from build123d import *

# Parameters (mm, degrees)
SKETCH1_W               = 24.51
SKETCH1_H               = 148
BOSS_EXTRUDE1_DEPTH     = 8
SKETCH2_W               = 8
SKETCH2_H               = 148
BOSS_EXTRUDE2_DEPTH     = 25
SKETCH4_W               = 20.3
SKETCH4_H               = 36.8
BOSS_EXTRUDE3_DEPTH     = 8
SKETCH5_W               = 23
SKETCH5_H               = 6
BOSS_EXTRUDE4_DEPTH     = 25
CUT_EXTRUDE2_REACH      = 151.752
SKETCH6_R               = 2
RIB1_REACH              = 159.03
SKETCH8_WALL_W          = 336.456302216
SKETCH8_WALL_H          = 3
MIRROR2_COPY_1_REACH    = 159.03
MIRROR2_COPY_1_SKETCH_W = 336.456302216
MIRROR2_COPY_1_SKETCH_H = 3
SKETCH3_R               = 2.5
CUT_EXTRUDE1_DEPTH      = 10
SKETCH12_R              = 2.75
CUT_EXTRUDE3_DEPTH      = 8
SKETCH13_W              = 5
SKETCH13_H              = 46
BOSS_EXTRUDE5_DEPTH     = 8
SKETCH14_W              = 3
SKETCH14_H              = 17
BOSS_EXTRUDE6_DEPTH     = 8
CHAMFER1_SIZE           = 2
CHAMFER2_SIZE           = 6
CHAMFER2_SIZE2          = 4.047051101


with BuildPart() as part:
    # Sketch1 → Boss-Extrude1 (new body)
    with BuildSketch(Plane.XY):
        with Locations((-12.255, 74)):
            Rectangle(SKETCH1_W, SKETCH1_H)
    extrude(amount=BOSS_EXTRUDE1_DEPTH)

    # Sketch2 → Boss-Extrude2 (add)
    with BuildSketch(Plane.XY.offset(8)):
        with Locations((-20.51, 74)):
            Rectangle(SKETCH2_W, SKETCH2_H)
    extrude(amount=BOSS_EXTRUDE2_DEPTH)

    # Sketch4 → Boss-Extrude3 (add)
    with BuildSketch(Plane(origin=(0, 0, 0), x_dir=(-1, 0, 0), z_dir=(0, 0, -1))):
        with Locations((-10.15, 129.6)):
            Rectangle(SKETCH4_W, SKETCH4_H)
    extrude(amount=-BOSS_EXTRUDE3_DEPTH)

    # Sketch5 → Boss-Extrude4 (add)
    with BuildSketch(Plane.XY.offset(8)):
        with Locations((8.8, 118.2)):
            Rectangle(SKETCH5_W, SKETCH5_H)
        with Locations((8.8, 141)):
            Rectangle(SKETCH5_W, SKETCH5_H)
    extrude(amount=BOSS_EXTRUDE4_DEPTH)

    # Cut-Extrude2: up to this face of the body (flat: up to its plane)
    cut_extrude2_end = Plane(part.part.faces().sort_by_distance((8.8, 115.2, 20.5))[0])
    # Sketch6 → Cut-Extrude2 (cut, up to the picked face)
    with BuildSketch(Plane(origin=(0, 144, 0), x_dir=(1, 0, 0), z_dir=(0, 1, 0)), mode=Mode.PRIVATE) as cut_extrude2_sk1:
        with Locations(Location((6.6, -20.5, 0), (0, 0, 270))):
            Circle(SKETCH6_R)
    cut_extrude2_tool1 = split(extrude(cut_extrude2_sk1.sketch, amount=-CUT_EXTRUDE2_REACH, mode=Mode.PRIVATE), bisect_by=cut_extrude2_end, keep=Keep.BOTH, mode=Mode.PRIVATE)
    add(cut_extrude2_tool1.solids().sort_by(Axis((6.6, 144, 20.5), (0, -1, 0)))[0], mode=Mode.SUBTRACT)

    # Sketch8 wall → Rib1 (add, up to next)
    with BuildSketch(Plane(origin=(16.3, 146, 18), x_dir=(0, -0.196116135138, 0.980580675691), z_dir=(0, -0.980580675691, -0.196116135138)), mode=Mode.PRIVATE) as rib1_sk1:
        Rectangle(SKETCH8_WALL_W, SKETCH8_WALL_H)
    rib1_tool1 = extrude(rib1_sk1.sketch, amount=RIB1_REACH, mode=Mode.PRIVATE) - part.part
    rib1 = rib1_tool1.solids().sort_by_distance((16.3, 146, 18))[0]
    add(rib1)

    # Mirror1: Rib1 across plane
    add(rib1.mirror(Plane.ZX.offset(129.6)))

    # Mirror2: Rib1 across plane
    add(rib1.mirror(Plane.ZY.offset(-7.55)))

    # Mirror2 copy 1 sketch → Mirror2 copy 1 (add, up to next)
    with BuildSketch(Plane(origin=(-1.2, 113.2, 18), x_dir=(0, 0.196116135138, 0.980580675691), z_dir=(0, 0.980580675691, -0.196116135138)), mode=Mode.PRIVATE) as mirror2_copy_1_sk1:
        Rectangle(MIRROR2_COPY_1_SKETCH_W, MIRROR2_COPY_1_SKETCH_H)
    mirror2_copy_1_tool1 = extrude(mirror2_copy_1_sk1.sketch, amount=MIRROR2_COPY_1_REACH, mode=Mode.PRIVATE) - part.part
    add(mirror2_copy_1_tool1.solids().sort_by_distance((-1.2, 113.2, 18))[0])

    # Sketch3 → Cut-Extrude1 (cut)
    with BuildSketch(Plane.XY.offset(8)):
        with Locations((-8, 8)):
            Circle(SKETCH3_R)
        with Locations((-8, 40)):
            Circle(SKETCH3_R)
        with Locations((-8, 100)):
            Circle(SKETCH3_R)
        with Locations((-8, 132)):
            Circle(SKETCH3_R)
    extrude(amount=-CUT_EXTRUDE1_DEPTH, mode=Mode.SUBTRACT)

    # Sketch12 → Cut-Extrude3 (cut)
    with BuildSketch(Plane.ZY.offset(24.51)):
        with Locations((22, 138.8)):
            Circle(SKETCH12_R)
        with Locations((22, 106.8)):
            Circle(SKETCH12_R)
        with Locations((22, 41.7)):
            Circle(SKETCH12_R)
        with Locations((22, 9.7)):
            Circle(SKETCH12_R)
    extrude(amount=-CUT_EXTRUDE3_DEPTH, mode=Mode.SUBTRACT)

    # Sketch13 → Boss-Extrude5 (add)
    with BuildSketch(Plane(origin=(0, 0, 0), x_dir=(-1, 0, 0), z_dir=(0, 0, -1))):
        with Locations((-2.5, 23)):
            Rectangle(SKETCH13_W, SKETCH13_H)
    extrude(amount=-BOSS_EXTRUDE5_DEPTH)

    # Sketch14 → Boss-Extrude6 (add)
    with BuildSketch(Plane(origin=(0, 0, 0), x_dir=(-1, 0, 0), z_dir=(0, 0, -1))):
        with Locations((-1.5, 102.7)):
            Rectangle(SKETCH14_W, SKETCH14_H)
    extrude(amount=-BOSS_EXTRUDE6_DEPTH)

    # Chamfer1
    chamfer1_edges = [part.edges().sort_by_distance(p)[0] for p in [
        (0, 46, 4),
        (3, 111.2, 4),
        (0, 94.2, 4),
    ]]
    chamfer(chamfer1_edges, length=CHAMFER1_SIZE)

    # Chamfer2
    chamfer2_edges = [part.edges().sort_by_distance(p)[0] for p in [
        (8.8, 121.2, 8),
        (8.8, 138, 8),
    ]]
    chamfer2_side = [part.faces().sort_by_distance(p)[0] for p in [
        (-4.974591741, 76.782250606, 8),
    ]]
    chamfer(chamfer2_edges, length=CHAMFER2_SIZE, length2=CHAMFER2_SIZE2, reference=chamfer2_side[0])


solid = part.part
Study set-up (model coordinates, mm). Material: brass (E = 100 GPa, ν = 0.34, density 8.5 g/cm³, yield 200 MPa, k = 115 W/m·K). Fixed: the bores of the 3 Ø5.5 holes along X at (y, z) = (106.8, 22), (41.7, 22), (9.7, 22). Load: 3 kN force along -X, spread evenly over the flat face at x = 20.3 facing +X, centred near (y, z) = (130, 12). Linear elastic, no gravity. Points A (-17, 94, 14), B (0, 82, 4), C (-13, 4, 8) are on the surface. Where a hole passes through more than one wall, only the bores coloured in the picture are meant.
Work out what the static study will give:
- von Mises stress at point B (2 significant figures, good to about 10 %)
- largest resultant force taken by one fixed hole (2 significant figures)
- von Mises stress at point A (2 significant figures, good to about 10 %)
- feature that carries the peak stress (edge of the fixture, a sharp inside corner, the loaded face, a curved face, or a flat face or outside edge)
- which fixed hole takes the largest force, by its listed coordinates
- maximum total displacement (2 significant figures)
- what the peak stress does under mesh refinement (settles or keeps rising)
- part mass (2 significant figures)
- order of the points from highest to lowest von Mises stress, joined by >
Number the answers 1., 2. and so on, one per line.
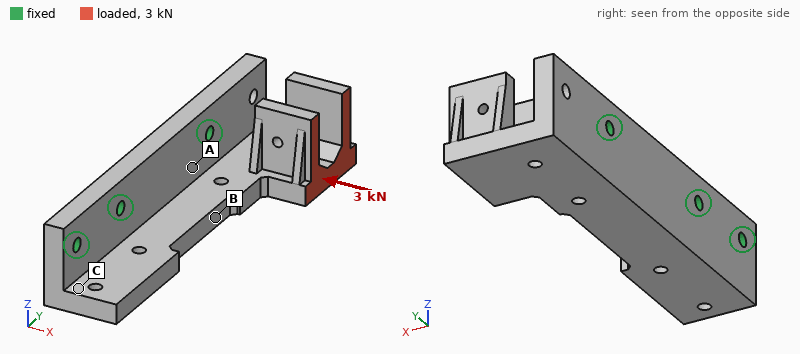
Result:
1. 34 MPa
2. 3.7 kN
3. 21 MPa
4. edge of the fixture
5. (106.8, 22)
6. 0.16 mm
7. keeps rising
8. 620 g
9. B > A > C
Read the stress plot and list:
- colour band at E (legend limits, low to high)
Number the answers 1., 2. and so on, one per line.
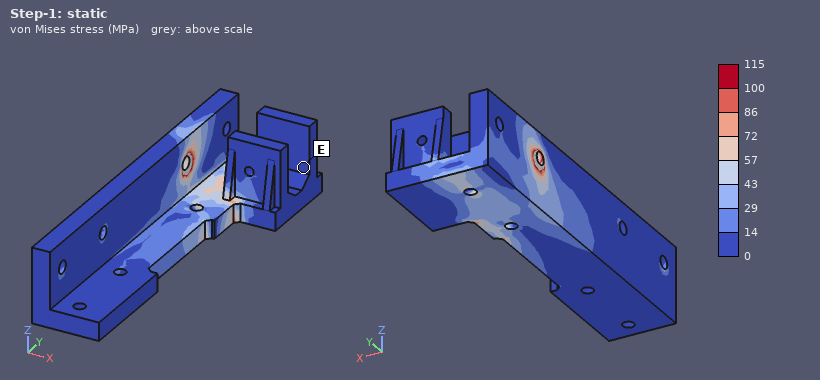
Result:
1. 0 to 14 MPa
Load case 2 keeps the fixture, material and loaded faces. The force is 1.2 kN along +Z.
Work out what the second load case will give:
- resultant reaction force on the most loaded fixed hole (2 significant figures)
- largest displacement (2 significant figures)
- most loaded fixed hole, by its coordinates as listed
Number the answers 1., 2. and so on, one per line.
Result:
1. 1.6 kN
2. 0.37 mm
3. (106.8, 22)
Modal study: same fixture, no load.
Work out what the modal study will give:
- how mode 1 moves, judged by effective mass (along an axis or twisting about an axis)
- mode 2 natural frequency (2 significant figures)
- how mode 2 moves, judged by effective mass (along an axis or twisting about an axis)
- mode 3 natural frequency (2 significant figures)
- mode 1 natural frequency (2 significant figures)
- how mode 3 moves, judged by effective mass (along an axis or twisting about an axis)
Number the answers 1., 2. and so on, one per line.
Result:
1. along Z
2. 1900 Hz
3. along X
4. 2700 Hz
5. 1100 Hz
6. along X
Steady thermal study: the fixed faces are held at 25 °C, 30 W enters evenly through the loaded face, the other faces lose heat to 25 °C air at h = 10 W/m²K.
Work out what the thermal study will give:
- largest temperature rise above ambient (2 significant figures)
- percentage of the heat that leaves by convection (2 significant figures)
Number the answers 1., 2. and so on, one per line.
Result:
1. 43 K
2. 9.5 %
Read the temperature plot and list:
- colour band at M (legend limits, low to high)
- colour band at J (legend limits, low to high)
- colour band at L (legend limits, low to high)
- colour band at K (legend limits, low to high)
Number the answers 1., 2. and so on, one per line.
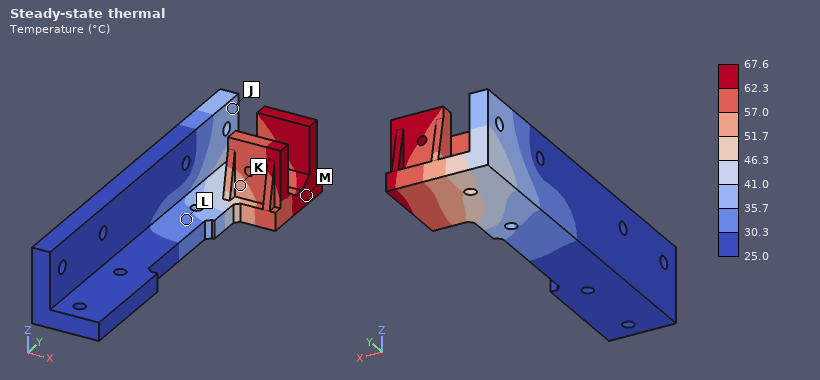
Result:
1. 62.3 to 67.6 °C
2. 35.7 to 41.0 °C
3. 30.3 to 35.7 °C
4. 51.7 to 57.0 °C
